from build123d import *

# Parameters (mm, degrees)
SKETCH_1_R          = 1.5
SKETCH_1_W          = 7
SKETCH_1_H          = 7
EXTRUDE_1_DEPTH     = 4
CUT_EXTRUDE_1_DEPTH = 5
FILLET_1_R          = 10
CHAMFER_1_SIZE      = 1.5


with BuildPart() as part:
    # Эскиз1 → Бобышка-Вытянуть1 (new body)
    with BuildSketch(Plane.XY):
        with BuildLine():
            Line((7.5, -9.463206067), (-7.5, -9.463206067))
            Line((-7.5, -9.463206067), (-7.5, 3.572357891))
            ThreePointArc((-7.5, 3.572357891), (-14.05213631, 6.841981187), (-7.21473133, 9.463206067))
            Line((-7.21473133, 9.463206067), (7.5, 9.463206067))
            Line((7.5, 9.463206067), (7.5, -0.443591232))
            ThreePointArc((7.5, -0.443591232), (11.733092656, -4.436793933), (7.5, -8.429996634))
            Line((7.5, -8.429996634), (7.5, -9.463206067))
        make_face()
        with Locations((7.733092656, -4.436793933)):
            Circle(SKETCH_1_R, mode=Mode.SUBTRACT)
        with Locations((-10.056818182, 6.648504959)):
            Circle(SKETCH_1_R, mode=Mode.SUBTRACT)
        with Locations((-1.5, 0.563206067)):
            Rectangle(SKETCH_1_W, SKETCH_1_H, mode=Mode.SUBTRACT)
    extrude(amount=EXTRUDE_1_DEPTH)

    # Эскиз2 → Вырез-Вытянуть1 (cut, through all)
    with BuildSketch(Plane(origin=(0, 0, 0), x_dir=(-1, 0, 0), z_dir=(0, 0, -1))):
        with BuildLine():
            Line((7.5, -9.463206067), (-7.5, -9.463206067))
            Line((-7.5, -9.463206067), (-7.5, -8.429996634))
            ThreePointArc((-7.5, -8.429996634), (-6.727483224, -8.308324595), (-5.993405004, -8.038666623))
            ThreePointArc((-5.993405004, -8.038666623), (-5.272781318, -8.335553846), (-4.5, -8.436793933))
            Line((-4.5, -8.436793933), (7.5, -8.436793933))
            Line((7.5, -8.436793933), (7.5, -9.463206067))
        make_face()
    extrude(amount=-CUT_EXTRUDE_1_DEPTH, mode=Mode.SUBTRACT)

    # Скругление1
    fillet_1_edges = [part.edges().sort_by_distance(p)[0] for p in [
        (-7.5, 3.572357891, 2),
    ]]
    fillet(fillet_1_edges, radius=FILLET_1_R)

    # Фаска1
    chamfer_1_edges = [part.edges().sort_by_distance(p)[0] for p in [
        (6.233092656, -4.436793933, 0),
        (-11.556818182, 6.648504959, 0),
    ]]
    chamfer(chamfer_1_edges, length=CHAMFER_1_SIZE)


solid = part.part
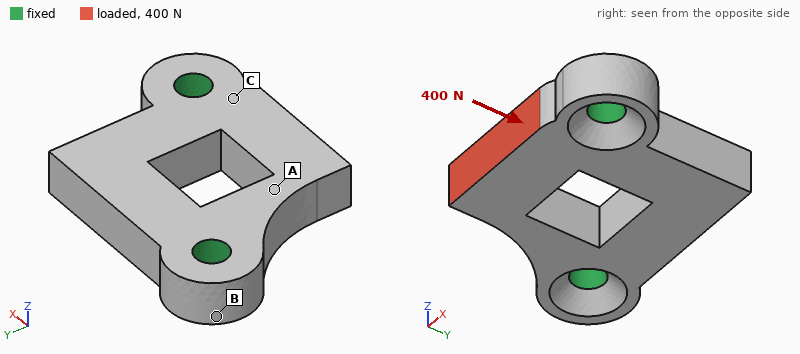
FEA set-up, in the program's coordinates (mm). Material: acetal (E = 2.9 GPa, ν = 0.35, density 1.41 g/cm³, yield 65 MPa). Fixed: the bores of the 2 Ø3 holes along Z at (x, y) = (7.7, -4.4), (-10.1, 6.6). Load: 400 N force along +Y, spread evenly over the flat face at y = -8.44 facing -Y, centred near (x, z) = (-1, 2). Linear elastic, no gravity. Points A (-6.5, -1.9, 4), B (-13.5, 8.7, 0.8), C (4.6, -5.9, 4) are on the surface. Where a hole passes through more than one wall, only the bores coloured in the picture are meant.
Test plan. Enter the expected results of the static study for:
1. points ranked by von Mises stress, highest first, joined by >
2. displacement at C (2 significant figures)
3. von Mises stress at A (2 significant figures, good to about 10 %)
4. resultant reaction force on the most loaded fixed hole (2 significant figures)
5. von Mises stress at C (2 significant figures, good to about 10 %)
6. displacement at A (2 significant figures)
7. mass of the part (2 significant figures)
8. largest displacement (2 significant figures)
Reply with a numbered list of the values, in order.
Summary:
1. A > C > B
2. 24 µm
3. 19 MPa
4. 210 N
5. 11 MPa
6. 43 µm
7. 1.6 g
8. 93 µm
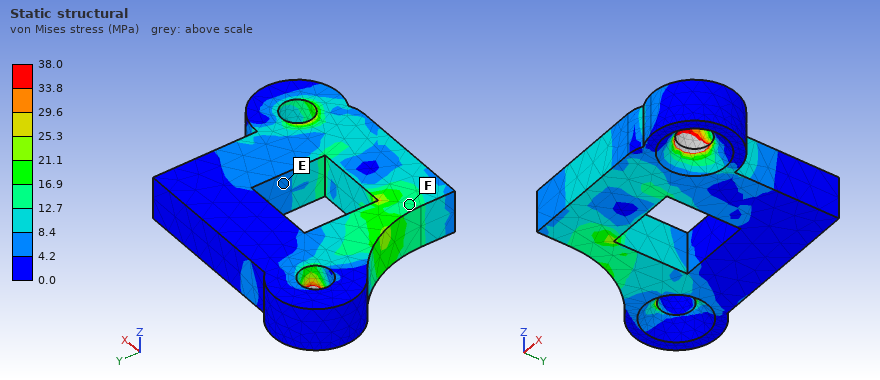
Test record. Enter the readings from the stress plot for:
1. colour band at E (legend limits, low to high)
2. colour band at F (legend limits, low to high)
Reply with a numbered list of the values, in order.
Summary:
1. 4.2 to 8.4 MPa
2. 12.7 to 16.9 MPa
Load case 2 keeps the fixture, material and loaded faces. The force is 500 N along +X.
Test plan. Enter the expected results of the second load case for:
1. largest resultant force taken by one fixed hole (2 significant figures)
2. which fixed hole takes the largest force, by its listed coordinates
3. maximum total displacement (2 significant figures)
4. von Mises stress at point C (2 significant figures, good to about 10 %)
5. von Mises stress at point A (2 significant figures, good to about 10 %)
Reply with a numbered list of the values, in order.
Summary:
1. 470 N
2. (7.7, -4.4)
3. 0.14 mm
4. 25 MPa
5. 14 MPa
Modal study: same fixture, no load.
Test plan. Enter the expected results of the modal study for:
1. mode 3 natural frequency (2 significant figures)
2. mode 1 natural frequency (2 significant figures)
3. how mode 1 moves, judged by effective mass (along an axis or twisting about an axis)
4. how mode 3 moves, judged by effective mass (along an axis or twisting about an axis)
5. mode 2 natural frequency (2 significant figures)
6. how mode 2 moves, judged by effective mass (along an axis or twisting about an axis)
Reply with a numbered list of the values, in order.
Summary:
1. 15 kHz
2. 5200 Hz
3. twisting about X
4. along Y
5. 6400 Hz
6. along Z
